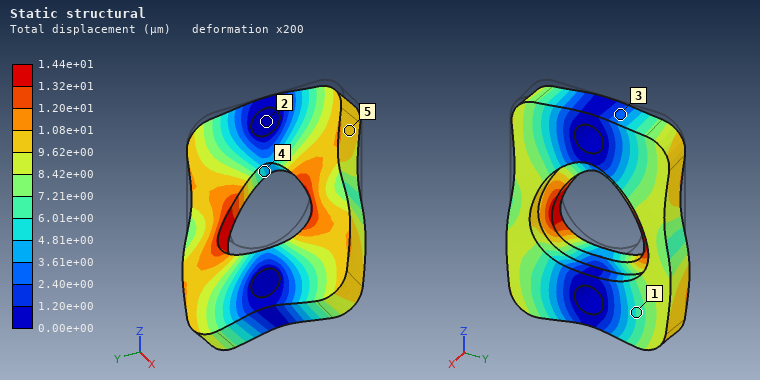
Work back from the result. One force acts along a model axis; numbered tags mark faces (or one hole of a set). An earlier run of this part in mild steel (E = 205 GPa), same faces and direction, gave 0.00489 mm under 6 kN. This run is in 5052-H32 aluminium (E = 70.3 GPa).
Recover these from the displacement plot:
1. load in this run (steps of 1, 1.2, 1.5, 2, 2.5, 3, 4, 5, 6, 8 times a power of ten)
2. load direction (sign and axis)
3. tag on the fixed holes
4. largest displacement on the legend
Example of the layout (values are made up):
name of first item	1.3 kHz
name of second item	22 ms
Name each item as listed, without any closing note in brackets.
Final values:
load in this run	6 kN
load direction	-Z
tag on the fixed holes	2
largest displacement on the legend	1.44e+01 µm
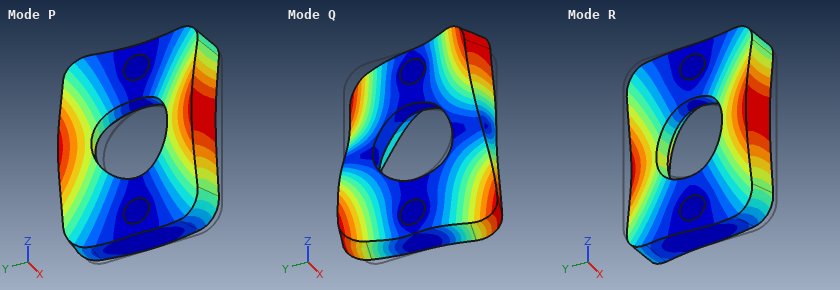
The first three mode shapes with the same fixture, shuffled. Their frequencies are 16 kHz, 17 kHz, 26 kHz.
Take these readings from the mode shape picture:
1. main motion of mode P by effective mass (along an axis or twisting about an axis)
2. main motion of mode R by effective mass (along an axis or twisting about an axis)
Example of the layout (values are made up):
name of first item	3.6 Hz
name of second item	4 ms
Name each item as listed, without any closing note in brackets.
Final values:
main motion of mode P by effective mass	along X
main motion of mode R by effective mass	twisting about Z
